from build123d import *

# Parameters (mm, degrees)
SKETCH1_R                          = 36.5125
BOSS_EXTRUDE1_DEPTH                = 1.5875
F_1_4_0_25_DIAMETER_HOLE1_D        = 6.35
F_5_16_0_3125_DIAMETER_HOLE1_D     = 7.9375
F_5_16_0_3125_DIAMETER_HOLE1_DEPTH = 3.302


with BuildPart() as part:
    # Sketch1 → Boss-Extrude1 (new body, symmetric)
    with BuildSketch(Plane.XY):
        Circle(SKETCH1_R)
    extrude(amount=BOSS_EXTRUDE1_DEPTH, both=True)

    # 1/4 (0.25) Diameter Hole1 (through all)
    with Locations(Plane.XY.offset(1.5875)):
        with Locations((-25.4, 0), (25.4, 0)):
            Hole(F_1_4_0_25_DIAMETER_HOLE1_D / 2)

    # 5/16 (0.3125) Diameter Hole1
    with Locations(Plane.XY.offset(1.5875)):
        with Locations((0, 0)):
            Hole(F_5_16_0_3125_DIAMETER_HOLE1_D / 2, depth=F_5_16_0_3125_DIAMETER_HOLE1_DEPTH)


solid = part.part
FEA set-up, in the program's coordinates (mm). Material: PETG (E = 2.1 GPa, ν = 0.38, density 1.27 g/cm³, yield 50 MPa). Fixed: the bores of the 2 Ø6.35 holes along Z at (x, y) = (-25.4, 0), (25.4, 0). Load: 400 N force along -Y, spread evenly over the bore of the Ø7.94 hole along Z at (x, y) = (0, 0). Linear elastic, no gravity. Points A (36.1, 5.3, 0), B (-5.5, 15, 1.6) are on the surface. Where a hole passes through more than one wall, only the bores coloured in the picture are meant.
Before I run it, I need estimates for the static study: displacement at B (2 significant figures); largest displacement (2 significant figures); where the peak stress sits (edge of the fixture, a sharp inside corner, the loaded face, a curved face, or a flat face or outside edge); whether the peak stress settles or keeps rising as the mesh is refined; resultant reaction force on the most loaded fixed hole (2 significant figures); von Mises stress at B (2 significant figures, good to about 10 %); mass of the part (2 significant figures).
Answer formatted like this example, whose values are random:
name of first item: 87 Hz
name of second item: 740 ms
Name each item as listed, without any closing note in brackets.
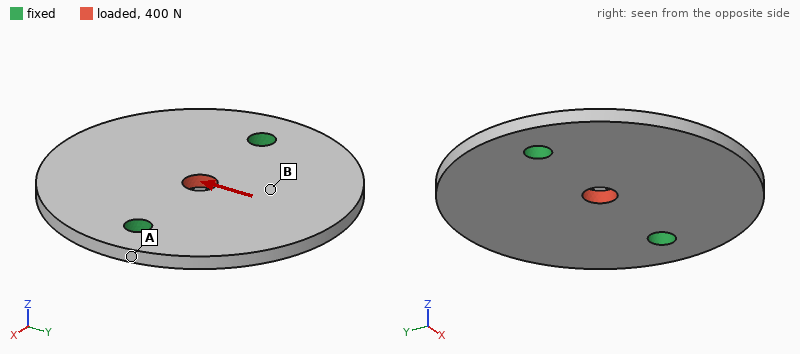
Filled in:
displacement at B: 38 µm
largest displacement: 59 µm
where the peak stress sits: edge of the fixture
whether the peak stress settles or keeps rising as the mesh is refined: keeps rising
resultant reaction force on the most loaded fixed hole: 200 N
von Mises stress at B: 2.2 MPa
mass of the part: 16 g
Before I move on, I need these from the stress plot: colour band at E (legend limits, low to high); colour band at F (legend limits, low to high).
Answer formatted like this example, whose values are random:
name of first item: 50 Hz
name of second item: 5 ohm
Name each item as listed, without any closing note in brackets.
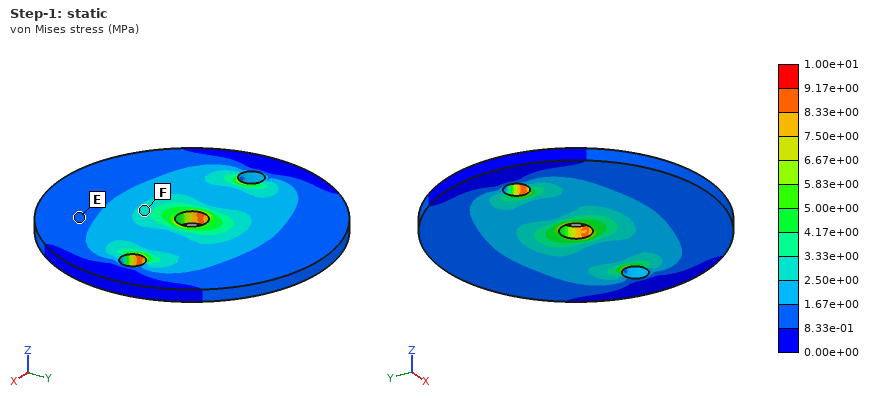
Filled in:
colour band at E: 8.33e-01 to 1.67e+00 MPa
colour band at F: 2.50e+00 to 3.33e+00 MPa
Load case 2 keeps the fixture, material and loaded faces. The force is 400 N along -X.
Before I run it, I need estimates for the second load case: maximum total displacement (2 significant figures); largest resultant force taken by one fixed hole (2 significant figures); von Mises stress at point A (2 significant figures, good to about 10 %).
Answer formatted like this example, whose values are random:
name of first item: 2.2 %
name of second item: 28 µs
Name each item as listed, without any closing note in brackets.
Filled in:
maximum total displacement: 41 µm
largest resultant force taken by one fixed hole: 200 N
von Mises stress at point A: 1.1 MPa
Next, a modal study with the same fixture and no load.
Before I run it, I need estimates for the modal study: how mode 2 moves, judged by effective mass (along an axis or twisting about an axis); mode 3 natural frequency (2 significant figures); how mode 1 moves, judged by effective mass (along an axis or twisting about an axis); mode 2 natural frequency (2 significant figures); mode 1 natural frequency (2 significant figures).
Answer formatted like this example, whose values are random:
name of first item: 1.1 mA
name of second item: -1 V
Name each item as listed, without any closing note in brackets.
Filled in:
how mode 2 moves, judged by effective mass: along Z
mode 3 natural frequency: 1400 Hz
how mode 1 moves, judged by effective mass: twisting about X
mode 2 natural frequency: 650 Hz
mode 1 natural frequency: 540 Hz
